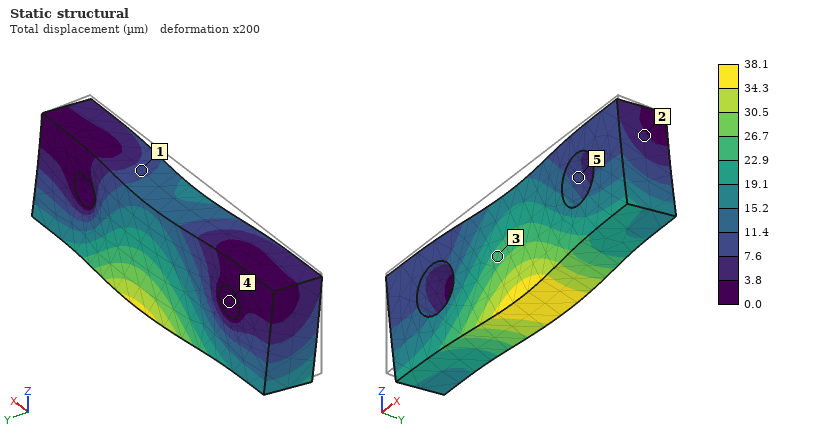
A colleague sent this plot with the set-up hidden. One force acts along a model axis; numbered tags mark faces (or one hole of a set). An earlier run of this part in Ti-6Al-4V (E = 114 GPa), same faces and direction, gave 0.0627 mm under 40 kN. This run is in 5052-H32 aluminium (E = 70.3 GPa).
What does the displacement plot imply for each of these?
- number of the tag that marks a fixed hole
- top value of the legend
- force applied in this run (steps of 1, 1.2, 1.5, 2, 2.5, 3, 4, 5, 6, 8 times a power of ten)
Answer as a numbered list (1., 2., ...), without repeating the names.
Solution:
1. 4
2. 38.1 µm
3. 15 kN
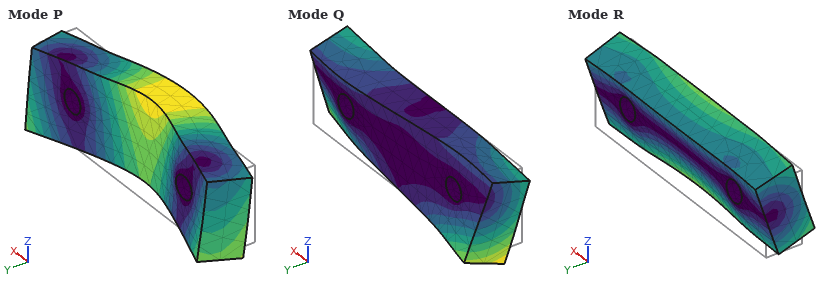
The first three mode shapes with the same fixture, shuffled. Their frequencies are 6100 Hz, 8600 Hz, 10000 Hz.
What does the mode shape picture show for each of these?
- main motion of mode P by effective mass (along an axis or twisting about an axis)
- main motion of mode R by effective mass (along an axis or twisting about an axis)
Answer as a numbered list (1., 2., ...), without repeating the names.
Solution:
1. along Y
2. along Z
